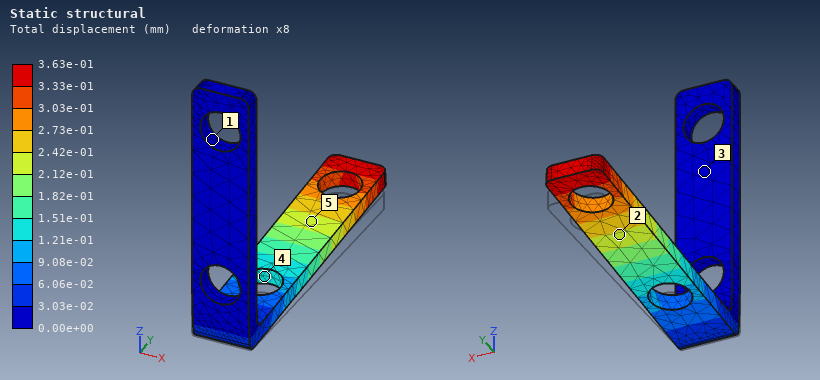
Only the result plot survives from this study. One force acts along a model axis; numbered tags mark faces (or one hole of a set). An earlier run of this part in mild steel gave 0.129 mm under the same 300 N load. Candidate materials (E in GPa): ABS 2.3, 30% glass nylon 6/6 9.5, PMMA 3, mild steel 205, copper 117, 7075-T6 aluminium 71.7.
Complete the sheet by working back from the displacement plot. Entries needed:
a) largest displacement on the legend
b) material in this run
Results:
3.63e-01 mm
7075-T6 aluminium
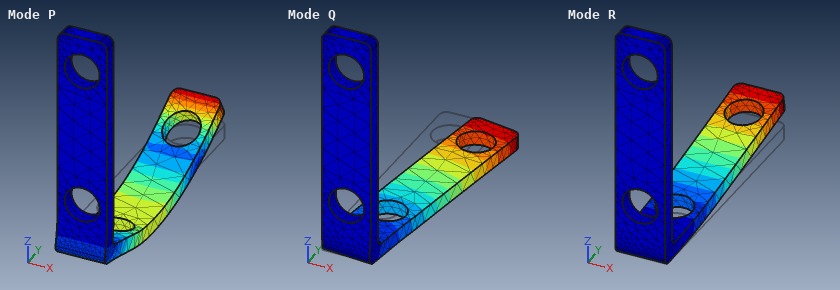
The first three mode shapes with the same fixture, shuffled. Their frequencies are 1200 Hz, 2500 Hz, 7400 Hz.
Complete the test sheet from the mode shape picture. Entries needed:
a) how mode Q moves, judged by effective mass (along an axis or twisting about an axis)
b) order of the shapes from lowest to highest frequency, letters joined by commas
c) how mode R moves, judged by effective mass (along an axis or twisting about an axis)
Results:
along X
R, Q, P
along Z
